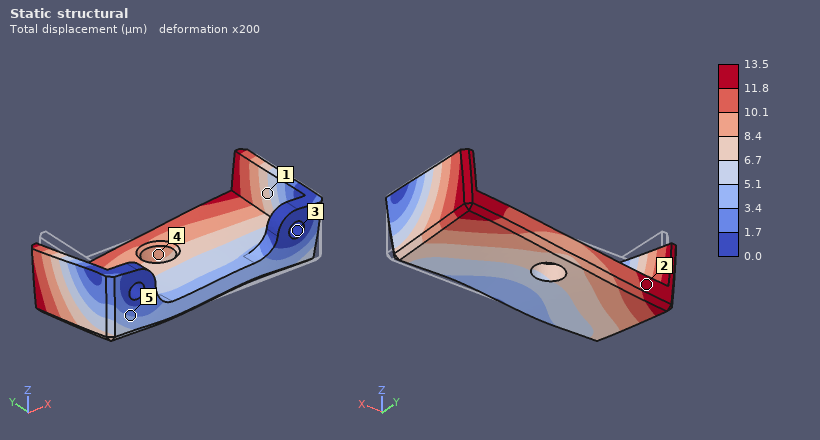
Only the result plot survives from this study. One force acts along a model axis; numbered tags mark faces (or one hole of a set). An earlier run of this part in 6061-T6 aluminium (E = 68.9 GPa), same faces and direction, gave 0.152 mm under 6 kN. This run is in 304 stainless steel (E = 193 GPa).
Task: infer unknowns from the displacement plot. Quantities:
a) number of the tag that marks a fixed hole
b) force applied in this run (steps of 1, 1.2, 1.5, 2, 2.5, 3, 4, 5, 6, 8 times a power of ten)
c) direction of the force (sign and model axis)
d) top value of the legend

3
1.5 kN
-X
13.5 µm
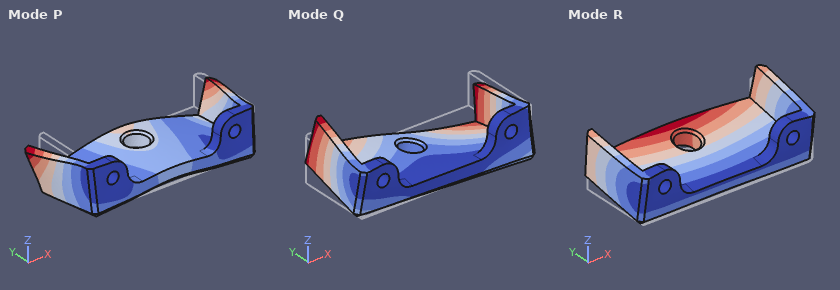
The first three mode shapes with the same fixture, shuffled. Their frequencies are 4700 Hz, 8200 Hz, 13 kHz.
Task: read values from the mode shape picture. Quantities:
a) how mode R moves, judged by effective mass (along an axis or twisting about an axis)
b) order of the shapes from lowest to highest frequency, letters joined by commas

along Z
R, Q, P
